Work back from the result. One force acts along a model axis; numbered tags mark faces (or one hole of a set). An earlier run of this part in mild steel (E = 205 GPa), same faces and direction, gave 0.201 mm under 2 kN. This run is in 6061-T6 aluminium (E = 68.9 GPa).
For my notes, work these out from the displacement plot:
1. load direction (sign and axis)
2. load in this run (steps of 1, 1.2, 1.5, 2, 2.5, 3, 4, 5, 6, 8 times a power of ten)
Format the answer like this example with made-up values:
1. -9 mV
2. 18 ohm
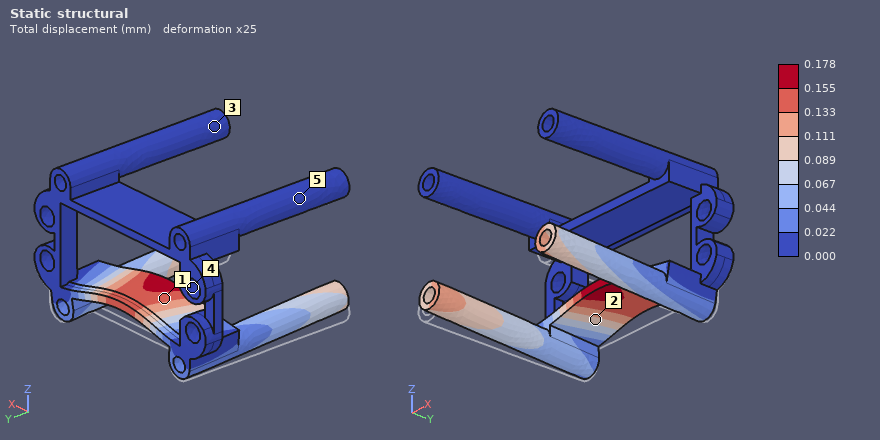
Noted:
1. +Z
2. 600 N
